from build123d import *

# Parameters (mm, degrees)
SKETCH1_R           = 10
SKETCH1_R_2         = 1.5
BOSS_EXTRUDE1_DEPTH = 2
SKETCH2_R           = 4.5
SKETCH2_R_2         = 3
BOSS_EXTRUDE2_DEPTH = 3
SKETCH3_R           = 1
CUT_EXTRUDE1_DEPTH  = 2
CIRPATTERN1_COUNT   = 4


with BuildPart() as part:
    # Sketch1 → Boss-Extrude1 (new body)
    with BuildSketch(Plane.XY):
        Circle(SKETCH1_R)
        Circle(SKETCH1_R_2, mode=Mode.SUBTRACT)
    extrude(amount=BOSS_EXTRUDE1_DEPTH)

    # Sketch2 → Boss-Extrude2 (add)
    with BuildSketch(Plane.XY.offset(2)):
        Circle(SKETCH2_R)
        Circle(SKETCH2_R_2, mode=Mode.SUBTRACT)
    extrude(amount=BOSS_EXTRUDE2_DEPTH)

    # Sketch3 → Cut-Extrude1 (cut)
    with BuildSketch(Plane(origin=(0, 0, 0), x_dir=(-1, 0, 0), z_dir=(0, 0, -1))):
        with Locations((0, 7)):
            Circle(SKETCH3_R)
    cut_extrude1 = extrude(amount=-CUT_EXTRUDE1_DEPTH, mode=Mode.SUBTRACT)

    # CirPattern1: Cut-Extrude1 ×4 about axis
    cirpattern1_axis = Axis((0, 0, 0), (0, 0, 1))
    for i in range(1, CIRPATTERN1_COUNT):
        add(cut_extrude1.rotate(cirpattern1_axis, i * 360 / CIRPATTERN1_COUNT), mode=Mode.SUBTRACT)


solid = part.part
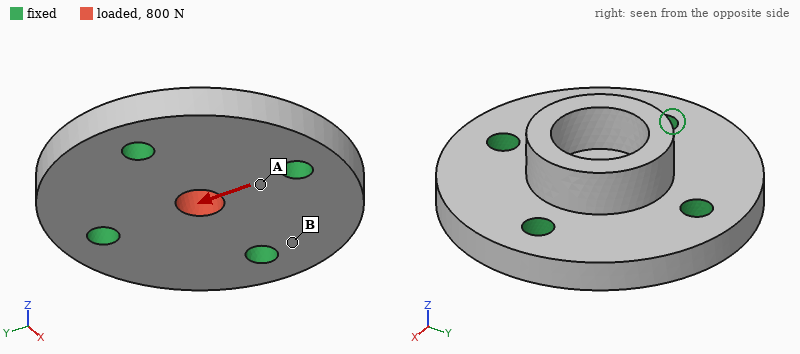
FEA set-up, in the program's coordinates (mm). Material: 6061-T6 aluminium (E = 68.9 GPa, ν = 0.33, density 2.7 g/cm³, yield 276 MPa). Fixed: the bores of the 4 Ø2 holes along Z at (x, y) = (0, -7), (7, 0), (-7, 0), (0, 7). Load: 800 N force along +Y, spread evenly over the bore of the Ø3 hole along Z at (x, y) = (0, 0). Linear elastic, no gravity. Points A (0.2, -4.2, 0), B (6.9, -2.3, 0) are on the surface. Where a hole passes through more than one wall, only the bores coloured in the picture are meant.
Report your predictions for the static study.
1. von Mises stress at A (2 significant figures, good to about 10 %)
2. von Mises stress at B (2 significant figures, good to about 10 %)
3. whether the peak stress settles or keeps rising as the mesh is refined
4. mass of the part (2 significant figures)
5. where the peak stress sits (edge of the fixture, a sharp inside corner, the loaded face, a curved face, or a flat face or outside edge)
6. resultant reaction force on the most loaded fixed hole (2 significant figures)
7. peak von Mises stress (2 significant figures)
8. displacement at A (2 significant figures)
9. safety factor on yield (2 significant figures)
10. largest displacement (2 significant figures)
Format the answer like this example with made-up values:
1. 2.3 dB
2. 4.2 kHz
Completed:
1. 40 MPa
2. 9.6 MPa
3. settles
4. 1.9 g
5. the loaded face
6. 270 N
7. 75 MPa
8. 1.1 µm
9. 3.7
10. 2.7 µm
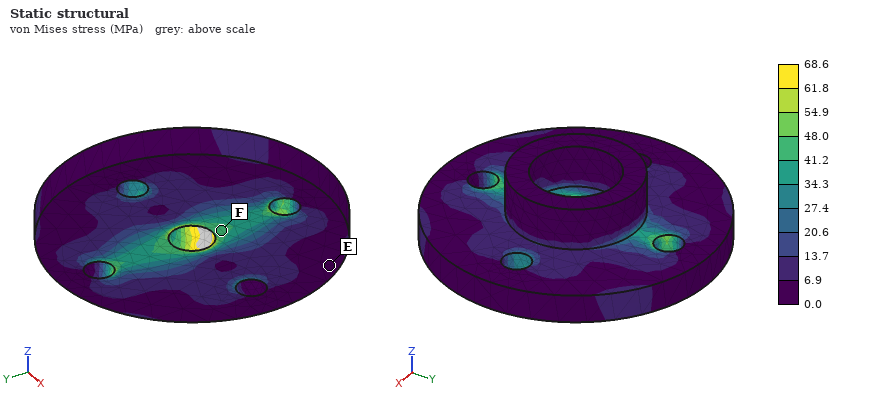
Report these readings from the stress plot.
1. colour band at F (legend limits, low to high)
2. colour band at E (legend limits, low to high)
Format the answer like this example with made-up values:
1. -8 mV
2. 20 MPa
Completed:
1. 41.2 to 48.0 MPa
2. 0.0 to 6.9 MPa
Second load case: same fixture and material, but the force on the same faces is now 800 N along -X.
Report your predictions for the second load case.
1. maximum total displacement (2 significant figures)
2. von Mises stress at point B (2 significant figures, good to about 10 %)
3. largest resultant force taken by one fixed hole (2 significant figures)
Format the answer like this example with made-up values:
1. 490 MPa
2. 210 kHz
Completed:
1. 2.7 µm
2. 13 MPa
3. 270 N
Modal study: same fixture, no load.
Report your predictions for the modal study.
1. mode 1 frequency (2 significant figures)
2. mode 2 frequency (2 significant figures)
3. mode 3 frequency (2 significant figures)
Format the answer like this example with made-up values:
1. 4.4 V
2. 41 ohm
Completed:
1. 62 kHz
2. 64 kHz
3. 64 kHz
